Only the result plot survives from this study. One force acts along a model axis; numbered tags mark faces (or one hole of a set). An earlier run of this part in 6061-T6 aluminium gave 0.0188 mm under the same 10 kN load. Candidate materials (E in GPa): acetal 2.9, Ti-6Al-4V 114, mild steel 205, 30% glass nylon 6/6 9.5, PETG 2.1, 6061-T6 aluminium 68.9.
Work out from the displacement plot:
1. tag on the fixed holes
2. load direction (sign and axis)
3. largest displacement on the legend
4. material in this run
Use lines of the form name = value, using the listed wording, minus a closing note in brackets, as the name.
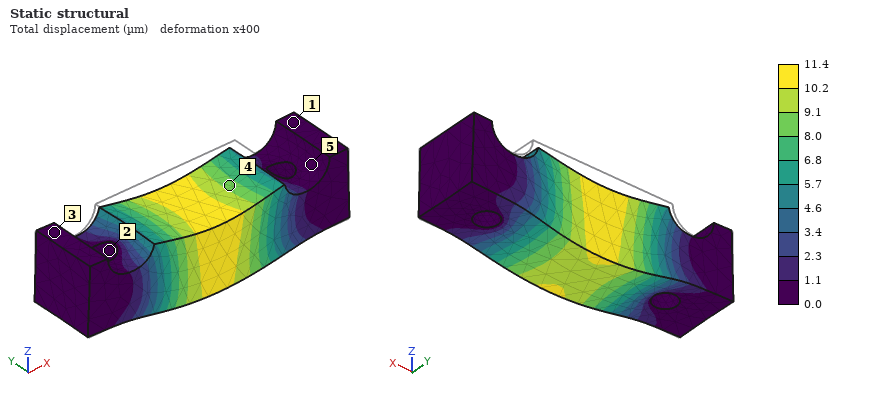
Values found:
tag on the fixed holes = 2
load direction = -Z
largest displacement on the legend = 11.4 µm
material in this run = Ti-6Al-4V
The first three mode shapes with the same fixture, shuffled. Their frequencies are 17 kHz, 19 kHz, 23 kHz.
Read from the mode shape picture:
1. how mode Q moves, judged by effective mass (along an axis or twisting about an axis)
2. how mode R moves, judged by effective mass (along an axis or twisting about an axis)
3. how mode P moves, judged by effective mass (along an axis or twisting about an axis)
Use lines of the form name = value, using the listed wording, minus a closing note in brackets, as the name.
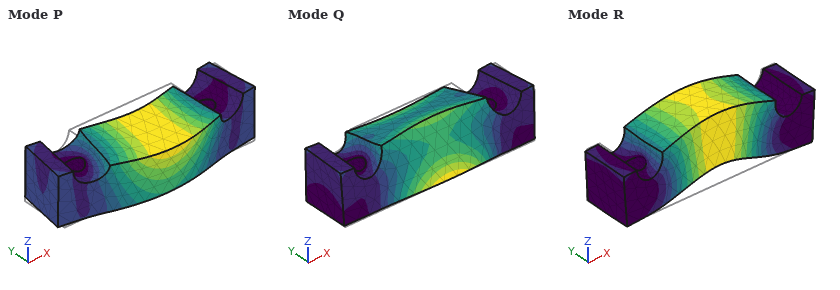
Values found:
how mode Q moves, judged by effective mass = twisting about X
how mode R moves, judged by effective mass = along Z
how mode P moves, judged by effective mass = along Y
